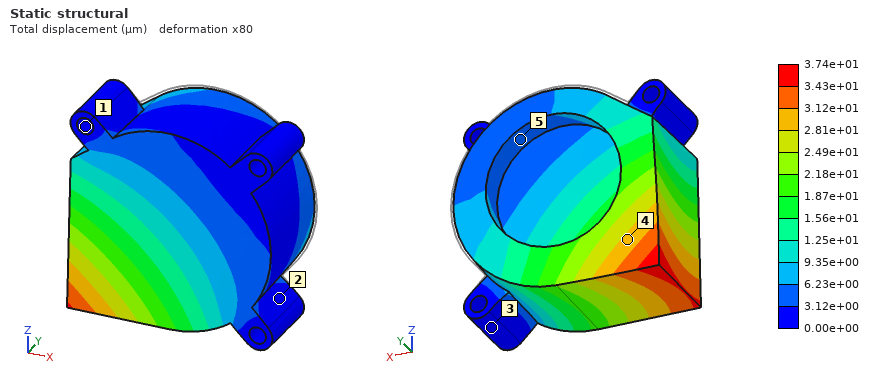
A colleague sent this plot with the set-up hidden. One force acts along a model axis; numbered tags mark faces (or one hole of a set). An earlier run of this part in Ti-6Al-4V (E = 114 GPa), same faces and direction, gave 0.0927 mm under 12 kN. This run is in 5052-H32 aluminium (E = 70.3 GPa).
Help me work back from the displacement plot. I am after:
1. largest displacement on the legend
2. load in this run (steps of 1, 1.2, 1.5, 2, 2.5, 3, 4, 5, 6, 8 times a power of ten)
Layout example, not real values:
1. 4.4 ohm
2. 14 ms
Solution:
1. 3.74e+01 µm
2. 3 kN
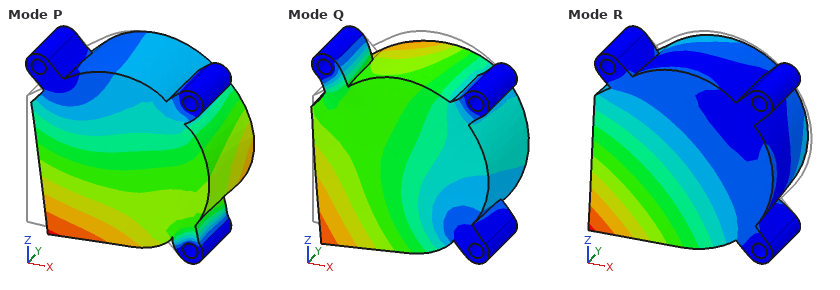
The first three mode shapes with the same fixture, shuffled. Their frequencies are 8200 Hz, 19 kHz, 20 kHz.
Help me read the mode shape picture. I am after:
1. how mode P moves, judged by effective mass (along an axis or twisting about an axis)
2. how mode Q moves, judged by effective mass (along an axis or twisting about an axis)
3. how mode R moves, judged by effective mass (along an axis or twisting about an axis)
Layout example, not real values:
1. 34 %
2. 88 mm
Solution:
1. along X
2. along Z
3. along Y
